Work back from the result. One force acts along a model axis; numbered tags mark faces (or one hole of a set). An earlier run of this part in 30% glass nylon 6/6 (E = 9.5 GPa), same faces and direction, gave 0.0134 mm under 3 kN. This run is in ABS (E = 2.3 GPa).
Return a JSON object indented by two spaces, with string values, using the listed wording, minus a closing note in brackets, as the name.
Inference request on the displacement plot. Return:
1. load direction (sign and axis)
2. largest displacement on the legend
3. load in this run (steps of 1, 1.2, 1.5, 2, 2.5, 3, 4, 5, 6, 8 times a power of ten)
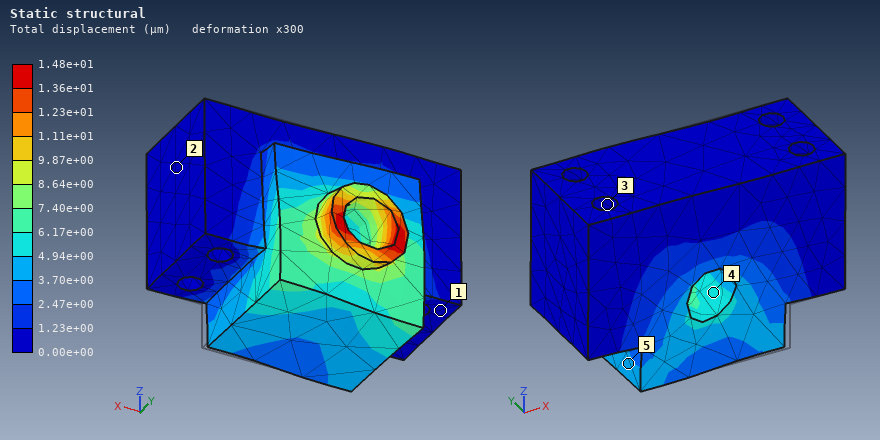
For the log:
{
  "load direction": "-X",
  "largest displacement on the legend": "1.48e+01 µm",
  "load in this run": "800 N"
}
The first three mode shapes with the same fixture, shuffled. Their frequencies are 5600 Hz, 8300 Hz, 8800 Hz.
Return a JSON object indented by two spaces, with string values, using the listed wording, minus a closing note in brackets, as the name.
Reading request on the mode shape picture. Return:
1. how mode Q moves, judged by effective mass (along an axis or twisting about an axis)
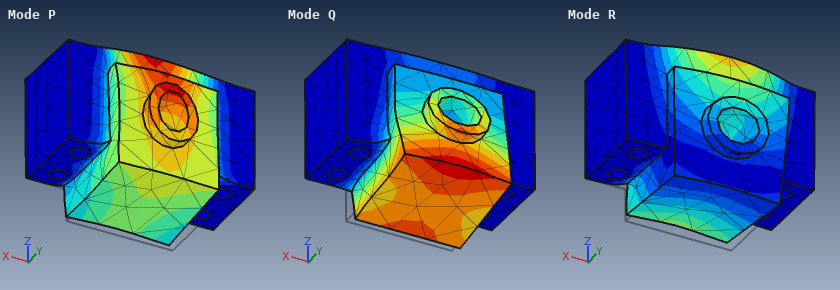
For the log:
{
  "how mode Q moves, judged by effective mass": "along Y"
}
